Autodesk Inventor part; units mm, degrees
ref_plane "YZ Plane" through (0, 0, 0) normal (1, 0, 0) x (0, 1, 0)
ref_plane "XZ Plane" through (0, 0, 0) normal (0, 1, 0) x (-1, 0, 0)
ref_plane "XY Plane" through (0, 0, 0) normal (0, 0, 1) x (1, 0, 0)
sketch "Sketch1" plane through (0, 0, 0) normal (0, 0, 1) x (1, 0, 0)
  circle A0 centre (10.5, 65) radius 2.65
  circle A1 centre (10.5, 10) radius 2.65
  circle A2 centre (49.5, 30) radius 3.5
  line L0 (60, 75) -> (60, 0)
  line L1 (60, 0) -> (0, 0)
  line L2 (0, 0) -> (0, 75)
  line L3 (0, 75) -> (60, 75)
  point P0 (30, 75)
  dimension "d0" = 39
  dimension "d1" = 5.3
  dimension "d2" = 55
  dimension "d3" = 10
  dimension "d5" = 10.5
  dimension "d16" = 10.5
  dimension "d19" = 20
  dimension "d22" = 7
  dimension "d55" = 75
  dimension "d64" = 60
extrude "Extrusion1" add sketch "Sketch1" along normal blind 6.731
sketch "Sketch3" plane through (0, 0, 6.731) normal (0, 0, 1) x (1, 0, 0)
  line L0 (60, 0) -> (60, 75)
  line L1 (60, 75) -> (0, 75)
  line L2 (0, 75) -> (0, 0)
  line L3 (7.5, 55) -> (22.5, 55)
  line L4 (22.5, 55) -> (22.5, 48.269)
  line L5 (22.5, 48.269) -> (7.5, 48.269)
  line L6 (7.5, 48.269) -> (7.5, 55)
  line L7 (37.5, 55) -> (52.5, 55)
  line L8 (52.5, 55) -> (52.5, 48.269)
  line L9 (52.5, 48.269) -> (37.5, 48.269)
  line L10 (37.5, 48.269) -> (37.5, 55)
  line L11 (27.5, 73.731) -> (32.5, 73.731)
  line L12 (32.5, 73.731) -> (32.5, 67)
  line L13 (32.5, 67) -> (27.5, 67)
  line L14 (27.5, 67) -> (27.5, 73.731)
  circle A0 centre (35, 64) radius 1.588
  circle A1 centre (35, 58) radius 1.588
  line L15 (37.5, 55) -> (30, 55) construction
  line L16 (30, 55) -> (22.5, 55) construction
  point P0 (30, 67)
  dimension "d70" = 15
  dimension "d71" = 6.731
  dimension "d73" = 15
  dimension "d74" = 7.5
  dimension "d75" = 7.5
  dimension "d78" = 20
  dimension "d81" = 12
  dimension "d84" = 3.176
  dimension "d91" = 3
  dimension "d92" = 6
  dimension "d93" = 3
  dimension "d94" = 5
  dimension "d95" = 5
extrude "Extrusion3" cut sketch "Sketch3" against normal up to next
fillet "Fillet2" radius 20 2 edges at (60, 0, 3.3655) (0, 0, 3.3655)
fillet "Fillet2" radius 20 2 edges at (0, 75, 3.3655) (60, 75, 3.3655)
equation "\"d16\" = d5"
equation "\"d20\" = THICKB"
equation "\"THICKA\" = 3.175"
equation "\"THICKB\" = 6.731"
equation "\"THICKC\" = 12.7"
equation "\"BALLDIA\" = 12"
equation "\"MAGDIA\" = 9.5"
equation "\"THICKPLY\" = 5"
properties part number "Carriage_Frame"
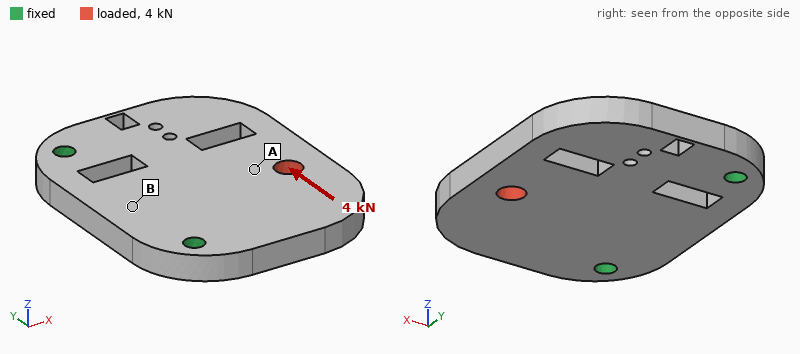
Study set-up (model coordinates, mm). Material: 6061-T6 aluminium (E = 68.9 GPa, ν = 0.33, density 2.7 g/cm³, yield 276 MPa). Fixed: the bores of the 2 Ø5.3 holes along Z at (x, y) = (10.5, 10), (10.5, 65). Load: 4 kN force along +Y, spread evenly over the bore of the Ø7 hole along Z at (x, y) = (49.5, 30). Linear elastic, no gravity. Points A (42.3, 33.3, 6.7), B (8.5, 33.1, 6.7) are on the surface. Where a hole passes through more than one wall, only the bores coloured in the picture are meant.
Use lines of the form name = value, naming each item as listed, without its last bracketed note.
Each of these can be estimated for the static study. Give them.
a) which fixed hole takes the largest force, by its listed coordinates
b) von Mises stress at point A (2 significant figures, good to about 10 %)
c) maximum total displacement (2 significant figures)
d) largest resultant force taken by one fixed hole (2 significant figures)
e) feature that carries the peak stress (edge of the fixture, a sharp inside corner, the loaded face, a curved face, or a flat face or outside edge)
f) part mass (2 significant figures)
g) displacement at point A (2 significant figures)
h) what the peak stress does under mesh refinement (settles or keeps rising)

which fixed hole takes the largest force, by its listed coordinates = (10.5, 10)
von Mises stress at point A = 31 MPa
maximum total displacement = 36 µm
largest resultant force taken by one fixed hole = 3.5 kN
feature that carries the peak stress = edge of the fixture
part mass = 69 g
displacement at point A = 24 µm
what the peak stress does under mesh refinement = keeps rising
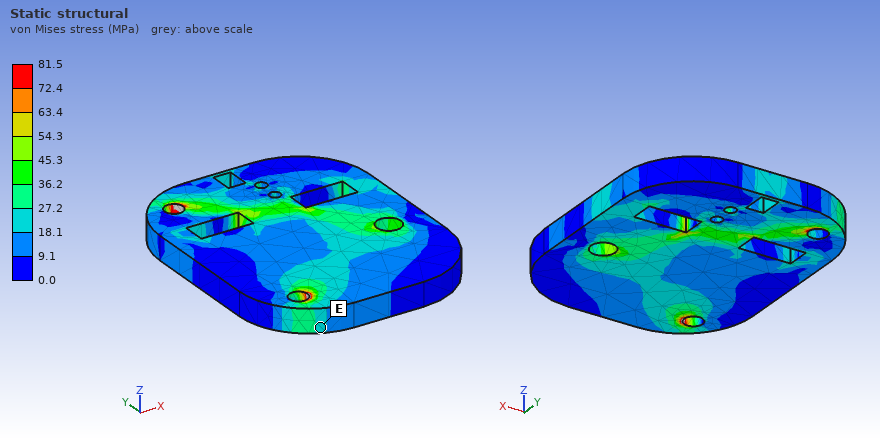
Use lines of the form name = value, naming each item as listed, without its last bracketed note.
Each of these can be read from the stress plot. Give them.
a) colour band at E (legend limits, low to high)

colour band at E = 18.1 to 27.2 MPa
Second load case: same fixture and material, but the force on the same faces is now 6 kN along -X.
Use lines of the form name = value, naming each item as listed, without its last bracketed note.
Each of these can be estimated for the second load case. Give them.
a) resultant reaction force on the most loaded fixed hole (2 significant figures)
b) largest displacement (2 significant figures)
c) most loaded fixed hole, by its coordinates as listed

resultant reaction force on the most loaded fixed hole = 3.9 kN
largest displacement = 27 µm
most loaded fixed hole, by its coordinates as listed = (10.5, 10)
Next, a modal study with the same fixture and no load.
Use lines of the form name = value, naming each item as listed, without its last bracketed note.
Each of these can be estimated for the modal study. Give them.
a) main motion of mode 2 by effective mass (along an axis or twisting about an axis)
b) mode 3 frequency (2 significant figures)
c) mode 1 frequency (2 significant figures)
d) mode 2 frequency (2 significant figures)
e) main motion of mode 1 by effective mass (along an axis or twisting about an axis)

main motion of mode 2 by effective mass = twisting about X
mode 3 frequency = 8400 Hz
mode 1 frequency = 2000 Hz
mode 2 frequency = 4400 Hz
main motion of mode 1 by effective mass = along Z
